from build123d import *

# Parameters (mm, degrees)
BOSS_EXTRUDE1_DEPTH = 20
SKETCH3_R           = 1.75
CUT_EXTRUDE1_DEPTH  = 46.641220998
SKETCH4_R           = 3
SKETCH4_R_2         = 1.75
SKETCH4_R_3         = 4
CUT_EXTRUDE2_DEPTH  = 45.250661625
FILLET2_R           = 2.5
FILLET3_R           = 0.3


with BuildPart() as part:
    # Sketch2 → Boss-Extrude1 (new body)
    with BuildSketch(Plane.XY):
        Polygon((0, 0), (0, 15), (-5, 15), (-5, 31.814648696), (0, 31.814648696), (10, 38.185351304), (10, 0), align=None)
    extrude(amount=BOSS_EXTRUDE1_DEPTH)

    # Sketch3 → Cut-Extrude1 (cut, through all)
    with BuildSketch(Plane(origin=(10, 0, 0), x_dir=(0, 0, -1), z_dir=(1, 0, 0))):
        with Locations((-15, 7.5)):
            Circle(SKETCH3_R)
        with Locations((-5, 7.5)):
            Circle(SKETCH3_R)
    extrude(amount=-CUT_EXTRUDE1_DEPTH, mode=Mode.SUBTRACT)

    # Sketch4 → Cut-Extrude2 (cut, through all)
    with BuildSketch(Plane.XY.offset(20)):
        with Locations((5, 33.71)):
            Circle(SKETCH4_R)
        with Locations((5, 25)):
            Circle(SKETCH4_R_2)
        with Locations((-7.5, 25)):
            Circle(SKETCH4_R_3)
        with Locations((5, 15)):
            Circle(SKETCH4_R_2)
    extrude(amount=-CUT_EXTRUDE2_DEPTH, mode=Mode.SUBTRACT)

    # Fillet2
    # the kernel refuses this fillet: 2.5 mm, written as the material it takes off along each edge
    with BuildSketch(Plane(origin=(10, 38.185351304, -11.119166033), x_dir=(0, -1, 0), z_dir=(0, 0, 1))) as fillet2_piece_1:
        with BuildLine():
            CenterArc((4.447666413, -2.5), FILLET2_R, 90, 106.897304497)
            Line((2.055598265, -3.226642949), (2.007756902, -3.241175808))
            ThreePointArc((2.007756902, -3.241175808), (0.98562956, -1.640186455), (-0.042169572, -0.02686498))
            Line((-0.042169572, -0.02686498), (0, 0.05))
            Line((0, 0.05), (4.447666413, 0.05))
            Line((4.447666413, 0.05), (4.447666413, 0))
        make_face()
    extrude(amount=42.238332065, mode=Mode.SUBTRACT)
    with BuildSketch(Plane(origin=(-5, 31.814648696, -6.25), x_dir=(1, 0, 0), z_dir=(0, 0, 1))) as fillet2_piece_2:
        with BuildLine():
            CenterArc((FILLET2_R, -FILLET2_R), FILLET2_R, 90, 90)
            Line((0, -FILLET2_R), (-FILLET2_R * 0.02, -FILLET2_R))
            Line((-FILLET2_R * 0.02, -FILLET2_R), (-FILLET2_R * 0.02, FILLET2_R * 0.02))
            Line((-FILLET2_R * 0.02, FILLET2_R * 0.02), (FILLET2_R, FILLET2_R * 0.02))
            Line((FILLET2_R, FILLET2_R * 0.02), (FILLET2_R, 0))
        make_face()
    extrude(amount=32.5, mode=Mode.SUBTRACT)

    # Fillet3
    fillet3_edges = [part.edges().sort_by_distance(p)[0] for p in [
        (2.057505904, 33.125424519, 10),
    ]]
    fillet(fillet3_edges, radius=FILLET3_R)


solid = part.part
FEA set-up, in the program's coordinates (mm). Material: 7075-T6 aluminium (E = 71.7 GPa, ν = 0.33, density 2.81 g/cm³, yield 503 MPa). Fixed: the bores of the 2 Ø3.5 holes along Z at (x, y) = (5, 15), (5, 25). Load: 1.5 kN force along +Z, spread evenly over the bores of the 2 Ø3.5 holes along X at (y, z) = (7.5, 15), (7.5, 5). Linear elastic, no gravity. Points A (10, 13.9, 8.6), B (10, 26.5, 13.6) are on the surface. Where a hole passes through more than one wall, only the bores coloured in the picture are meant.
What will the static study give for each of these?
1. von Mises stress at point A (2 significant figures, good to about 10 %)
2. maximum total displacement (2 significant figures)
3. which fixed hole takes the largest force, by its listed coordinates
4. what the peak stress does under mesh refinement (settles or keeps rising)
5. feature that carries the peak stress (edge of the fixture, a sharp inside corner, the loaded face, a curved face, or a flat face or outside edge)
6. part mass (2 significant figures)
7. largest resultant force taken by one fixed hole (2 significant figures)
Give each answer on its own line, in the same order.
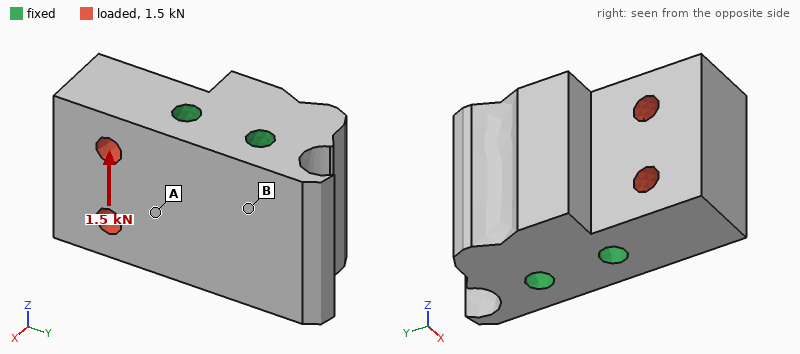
6.7 MPa
4.0 µm
(5, 15)
keeps rising
edge of the fixture
21 g
1.5 kN
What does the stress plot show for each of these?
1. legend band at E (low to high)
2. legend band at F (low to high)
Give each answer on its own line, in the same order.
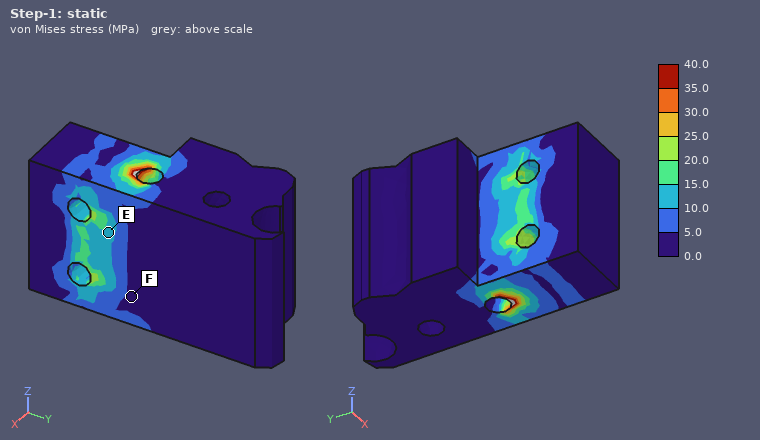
10.0 to 15.0 MPa
0.0 to 5.0 MPa
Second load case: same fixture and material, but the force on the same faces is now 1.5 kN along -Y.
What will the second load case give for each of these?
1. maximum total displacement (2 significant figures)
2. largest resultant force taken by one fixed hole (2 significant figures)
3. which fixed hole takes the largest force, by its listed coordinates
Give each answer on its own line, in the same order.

1.2 µm
1.3 kN
(5, 15)
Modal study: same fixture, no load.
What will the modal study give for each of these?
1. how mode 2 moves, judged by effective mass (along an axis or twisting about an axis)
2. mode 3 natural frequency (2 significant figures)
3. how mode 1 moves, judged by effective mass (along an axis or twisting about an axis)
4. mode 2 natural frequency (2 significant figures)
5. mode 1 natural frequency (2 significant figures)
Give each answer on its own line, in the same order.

along Z
40 kHz
along X
37 kHz
24 kHz
